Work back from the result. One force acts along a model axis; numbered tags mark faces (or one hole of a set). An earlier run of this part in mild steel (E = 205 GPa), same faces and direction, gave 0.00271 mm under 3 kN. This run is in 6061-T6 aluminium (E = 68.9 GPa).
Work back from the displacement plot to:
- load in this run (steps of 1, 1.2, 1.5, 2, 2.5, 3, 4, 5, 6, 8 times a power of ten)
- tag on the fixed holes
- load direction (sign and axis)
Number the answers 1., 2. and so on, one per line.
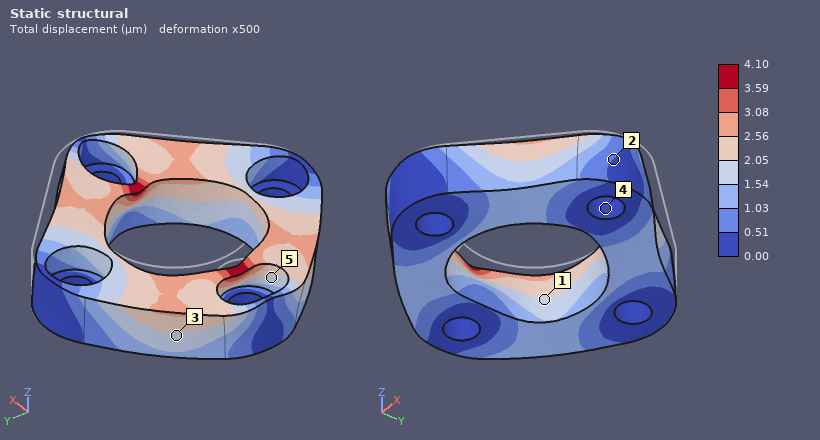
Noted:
1. 1.5 kN
2. 4
3. -X
